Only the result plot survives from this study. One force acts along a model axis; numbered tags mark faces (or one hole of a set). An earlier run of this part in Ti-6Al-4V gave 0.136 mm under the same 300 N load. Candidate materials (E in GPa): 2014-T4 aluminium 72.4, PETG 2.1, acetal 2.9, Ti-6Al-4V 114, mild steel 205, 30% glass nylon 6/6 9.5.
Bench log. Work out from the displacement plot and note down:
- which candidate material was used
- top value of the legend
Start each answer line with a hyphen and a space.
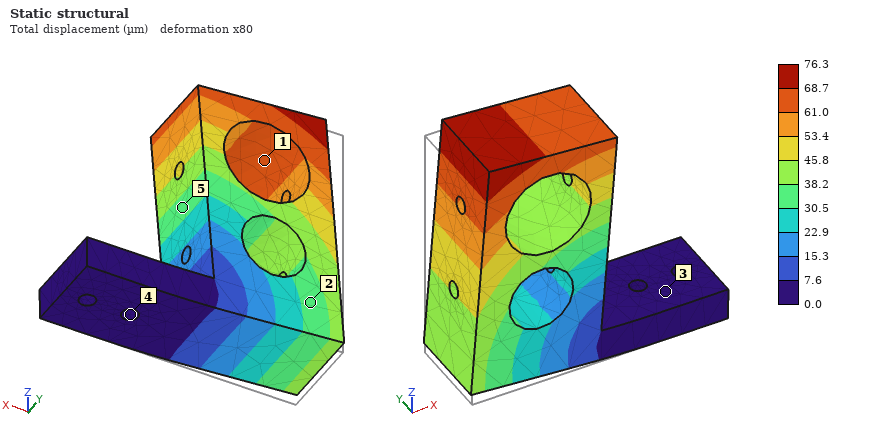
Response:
- mild steel
- 76.3 µm
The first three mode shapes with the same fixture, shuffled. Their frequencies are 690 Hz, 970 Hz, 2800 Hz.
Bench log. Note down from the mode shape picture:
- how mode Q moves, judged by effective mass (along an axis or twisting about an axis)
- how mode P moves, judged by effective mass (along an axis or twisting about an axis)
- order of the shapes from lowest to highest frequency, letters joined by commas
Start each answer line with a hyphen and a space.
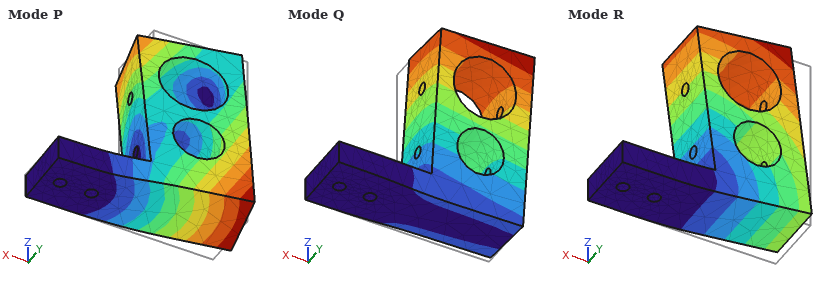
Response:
- along Y
- along Y
- R, Q, P
